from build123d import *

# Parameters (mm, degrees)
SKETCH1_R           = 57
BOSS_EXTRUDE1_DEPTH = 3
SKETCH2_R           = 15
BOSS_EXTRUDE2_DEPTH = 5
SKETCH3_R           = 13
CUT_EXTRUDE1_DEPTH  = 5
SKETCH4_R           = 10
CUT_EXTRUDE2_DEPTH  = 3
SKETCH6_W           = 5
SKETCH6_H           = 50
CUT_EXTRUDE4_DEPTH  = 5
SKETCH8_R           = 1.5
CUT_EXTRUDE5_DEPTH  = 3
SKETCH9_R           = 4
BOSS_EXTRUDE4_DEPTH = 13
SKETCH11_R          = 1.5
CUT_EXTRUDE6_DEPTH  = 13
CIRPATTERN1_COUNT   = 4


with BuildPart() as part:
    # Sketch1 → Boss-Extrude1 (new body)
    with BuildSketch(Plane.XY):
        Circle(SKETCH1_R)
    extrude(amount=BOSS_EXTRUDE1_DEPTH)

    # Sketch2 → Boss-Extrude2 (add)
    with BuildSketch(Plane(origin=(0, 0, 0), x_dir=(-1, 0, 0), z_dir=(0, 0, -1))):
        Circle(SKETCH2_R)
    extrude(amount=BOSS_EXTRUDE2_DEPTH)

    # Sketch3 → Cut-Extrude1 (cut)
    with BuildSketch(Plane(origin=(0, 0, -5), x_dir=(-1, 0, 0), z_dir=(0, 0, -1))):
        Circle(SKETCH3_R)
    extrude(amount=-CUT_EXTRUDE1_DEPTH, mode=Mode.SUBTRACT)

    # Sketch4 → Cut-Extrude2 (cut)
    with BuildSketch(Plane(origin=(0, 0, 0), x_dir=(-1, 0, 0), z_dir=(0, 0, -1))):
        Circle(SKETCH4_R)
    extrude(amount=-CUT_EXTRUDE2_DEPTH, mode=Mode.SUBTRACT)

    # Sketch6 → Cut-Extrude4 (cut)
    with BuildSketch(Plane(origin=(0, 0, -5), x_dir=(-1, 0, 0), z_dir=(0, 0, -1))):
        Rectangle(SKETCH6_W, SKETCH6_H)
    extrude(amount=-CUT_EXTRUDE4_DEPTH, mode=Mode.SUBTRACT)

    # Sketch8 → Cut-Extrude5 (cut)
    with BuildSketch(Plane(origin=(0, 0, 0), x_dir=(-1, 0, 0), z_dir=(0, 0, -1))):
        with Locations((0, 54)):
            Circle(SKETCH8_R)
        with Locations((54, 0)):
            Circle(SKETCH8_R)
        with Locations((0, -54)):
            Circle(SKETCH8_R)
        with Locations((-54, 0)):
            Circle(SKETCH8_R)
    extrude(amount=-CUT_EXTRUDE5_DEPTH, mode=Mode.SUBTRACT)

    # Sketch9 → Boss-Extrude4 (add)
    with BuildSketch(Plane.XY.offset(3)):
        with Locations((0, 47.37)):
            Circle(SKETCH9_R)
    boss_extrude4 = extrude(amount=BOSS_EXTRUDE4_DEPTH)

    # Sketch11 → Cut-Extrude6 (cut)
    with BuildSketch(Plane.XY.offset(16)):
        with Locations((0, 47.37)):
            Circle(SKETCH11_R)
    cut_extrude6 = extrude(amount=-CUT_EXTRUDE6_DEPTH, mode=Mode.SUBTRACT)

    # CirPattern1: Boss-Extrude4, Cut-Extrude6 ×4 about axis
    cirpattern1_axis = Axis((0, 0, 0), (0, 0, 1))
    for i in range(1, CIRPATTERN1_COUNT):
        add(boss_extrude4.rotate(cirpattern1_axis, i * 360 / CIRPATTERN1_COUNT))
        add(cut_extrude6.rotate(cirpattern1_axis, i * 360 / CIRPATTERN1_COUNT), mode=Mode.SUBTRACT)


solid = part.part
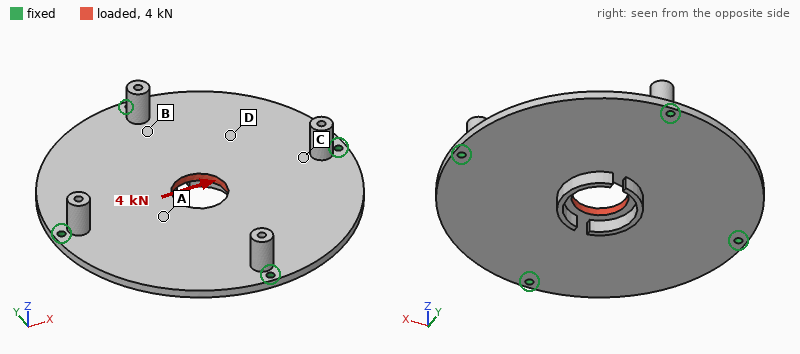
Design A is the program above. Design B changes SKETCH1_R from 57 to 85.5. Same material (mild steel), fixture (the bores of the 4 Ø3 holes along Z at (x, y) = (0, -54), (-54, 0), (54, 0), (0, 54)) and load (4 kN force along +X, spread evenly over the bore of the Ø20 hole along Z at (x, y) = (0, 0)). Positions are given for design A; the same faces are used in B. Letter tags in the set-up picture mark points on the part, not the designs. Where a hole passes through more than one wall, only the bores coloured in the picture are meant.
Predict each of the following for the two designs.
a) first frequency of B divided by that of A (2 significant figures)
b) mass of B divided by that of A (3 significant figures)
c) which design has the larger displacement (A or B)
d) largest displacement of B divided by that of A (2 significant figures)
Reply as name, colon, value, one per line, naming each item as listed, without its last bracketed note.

first frequency of B divided by that of A: 0.52
mass of B divided by that of A: 2.17
which design has the larger displacement: A
largest displacement of B divided by that of A: 0.80
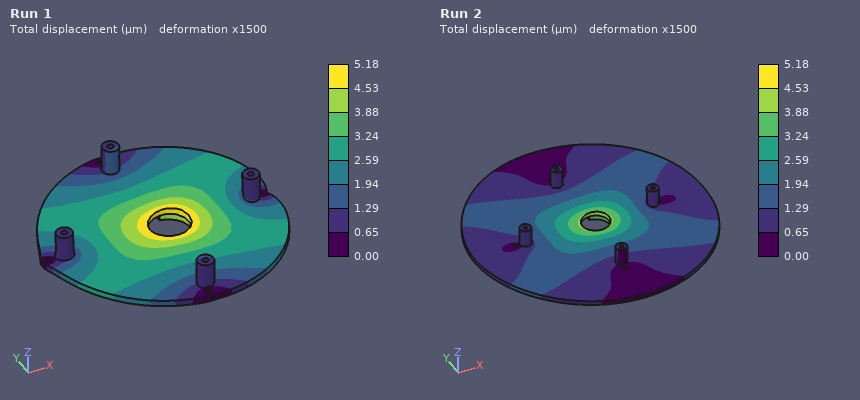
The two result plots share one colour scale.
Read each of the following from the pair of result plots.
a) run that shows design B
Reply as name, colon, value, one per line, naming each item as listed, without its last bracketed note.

run that shows design B: Run 2
